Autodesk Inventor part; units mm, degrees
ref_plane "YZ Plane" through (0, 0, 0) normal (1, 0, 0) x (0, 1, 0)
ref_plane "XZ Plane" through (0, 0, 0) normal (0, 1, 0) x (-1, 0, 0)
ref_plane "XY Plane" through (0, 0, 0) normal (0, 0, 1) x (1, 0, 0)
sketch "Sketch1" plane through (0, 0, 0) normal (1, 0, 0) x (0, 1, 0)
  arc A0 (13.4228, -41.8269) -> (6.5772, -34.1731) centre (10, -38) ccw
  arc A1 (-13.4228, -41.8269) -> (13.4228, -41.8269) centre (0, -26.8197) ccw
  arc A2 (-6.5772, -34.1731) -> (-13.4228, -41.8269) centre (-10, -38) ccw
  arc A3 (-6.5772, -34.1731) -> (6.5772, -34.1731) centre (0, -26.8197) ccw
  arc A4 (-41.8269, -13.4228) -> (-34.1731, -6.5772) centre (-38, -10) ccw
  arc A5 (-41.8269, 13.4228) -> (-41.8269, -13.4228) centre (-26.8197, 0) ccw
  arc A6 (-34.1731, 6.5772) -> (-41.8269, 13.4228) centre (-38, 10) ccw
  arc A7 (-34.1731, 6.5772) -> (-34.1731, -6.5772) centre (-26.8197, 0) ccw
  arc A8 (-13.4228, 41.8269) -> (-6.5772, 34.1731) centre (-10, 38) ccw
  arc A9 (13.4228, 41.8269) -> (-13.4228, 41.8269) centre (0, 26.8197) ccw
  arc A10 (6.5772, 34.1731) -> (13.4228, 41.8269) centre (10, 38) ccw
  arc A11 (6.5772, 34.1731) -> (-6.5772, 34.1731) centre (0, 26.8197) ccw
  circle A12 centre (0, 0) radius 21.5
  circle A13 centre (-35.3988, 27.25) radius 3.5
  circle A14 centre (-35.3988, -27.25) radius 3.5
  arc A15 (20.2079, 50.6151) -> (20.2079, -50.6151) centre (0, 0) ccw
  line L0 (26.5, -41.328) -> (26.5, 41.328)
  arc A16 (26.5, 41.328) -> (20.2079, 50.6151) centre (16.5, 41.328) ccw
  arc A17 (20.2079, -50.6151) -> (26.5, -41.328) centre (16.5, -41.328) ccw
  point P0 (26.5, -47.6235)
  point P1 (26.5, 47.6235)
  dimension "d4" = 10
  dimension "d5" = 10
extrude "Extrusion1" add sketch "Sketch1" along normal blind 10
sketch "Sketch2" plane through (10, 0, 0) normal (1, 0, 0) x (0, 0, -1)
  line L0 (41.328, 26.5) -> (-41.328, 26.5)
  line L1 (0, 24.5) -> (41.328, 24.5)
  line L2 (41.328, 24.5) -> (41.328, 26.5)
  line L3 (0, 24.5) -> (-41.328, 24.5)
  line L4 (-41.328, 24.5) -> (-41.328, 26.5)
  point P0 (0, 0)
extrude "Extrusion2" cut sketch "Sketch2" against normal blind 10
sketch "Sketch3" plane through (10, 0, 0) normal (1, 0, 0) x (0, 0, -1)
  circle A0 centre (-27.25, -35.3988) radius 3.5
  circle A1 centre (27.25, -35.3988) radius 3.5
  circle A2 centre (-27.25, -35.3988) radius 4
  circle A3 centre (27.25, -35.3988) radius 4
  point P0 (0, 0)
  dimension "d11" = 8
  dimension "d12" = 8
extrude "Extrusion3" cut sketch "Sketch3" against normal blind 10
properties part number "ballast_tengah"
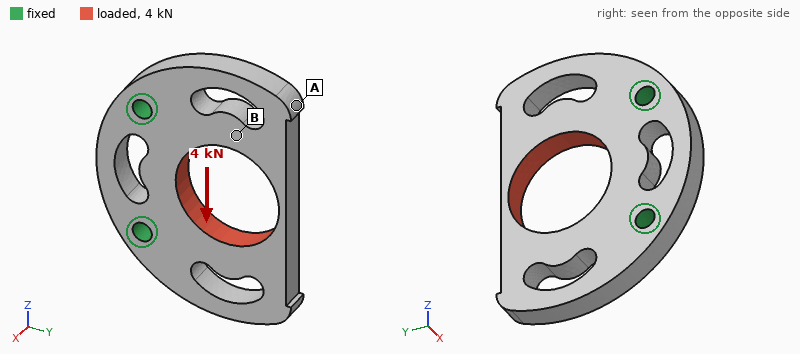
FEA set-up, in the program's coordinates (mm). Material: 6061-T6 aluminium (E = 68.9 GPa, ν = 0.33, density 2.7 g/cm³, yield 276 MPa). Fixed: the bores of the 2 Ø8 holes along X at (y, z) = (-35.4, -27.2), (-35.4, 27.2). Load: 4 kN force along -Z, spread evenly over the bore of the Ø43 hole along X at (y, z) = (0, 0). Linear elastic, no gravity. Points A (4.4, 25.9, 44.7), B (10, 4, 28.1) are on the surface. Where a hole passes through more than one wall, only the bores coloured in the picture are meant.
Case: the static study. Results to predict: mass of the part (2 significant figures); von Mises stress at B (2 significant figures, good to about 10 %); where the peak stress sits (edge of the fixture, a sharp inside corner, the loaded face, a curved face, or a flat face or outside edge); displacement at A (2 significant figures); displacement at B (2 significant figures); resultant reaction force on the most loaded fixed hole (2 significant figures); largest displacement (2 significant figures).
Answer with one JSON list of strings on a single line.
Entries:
["130 g", "16 MPa", "edge of the fixture", "77 µm", "46 µm", "2.6 kN", "77 µm"]
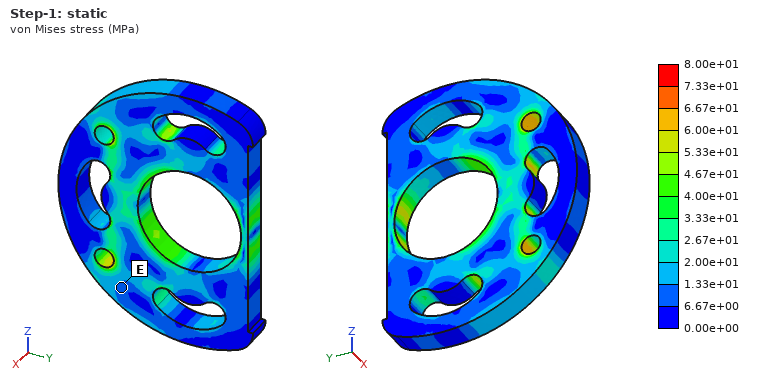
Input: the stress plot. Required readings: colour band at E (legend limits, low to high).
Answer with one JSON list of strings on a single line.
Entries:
["6.67e+00 to 1.33e+01 MPa"]
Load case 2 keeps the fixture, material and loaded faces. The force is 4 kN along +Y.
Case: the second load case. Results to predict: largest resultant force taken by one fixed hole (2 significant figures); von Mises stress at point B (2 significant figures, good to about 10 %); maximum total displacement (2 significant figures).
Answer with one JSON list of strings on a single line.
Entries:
["2.0 kN", "7.5 MPa", "28 µm"]
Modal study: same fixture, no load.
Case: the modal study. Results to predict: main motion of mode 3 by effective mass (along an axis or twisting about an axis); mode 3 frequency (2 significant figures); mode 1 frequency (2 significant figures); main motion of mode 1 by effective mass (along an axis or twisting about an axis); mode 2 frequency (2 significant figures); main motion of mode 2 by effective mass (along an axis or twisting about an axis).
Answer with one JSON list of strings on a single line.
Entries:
["along Z", "4400 Hz", "2000 Hz", "along X", "2700 Hz", "twisting about Y"]
